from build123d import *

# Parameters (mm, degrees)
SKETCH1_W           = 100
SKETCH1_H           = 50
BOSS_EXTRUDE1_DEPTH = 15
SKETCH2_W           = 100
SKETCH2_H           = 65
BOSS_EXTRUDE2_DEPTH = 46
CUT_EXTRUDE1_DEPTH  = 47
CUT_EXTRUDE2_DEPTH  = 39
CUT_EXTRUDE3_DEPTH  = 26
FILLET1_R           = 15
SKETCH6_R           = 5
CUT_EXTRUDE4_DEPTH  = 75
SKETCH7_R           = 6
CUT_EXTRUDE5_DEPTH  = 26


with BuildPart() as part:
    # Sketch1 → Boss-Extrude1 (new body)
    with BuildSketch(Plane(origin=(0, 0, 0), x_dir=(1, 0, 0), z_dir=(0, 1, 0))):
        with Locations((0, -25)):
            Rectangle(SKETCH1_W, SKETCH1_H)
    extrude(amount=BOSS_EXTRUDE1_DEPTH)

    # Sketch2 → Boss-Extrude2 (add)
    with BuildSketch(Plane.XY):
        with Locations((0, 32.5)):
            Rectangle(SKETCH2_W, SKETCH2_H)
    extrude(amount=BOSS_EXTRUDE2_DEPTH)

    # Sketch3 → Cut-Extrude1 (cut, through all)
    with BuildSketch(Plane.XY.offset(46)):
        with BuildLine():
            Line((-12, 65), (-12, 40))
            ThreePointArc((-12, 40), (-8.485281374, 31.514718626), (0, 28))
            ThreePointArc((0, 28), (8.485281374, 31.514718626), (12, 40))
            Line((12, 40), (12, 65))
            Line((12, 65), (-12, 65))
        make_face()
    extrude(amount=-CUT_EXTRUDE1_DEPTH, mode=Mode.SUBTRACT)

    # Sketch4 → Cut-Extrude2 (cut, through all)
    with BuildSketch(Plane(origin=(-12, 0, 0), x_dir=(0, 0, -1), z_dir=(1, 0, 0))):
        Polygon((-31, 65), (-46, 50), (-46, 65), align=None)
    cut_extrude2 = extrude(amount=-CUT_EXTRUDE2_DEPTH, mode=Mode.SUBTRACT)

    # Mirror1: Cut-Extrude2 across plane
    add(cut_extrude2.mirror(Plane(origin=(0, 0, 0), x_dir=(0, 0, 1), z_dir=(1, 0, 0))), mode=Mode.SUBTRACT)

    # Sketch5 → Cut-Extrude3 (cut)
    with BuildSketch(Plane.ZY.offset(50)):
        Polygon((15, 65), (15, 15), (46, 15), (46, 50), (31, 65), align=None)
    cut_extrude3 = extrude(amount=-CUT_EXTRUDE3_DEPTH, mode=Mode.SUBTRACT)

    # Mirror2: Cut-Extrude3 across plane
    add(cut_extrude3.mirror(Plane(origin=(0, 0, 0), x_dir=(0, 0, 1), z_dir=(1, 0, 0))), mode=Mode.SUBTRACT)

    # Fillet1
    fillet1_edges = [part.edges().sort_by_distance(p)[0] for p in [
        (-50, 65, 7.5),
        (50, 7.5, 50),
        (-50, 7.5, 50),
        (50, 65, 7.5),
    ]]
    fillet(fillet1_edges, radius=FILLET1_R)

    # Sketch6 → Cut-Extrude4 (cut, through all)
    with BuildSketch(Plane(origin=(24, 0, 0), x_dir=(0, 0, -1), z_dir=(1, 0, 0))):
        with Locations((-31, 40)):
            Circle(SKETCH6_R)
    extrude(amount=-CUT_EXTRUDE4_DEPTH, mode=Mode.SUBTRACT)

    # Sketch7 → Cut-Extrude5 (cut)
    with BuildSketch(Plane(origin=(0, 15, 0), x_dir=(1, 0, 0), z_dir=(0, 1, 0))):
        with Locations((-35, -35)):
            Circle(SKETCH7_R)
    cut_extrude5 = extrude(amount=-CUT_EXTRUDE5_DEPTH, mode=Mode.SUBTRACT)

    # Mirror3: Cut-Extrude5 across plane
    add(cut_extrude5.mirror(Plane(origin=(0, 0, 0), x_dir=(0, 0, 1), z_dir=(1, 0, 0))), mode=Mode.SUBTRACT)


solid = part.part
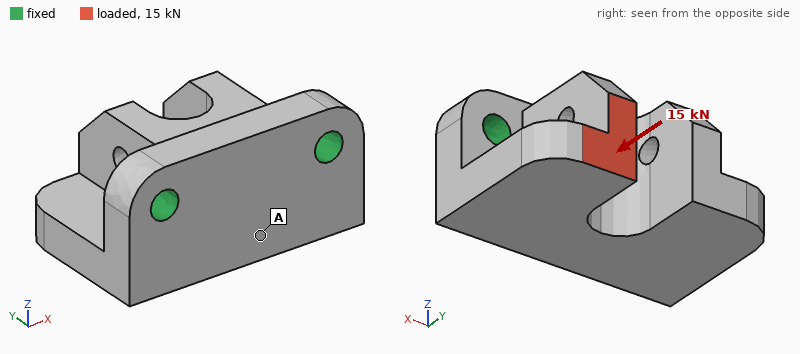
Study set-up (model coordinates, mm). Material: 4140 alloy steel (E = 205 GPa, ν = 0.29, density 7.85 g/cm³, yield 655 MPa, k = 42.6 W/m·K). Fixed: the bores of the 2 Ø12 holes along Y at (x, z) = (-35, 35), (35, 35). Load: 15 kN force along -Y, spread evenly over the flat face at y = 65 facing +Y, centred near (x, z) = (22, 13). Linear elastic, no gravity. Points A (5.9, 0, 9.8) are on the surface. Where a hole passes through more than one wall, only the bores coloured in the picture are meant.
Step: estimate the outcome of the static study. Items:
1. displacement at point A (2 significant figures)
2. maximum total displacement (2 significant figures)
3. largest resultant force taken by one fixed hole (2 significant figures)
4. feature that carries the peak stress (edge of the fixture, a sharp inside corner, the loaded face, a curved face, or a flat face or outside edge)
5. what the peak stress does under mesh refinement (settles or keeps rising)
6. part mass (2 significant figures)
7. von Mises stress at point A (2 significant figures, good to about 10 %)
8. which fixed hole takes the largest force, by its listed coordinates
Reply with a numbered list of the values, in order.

1. 18 µm
2. 50 µm
3. 12 kN
4. edge of the fixture
5. keeps rising
6. 1.4 kg
7. 21 MPa
8. (35, 35)
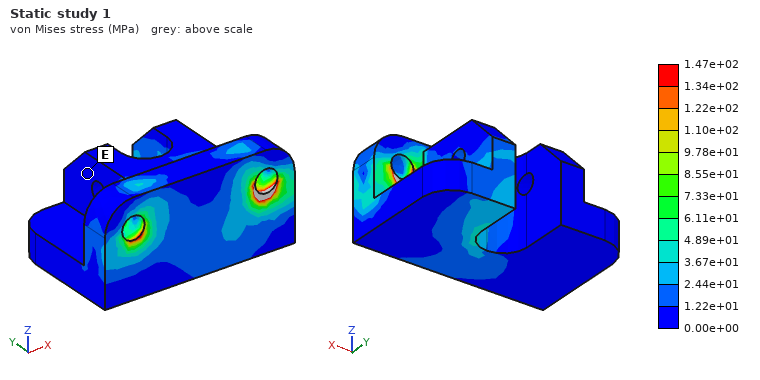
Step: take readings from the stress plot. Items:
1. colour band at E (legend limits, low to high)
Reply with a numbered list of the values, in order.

1. 0.00e+00 to 1.22e+01 MPa
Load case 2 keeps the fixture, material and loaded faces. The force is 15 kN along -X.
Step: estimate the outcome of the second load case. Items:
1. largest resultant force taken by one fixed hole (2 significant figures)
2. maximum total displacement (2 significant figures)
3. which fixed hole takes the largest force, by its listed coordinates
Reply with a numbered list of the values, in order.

1. 17 kN
2. 93 µm
3. (-35, 35)
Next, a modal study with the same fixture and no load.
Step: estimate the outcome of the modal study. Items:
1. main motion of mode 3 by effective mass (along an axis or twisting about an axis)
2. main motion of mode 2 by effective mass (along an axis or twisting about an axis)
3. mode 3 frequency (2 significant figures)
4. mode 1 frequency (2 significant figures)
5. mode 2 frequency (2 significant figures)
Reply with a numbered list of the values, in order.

1. along X
2. along X
3. 6800 Hz
4. 2900 Hz
5. 5700 Hz
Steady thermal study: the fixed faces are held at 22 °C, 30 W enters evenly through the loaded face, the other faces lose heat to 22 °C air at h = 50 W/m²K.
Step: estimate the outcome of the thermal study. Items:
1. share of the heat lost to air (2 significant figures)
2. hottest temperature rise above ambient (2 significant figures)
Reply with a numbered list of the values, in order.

1. 40 %
2. 46 K
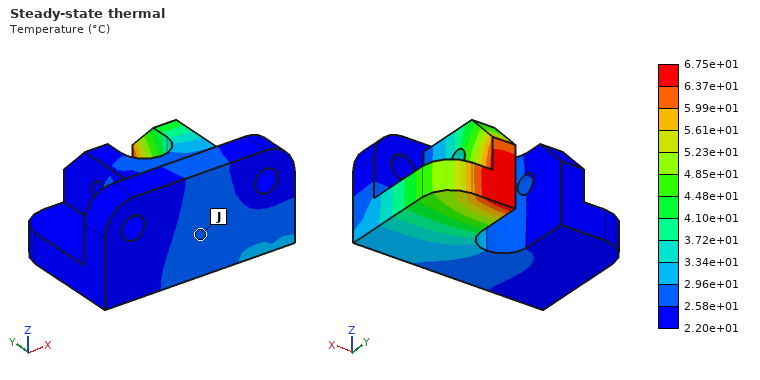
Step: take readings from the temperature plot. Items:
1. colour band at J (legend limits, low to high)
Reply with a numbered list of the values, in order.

1. 2.58e+01 to 2.96e+01 °C
